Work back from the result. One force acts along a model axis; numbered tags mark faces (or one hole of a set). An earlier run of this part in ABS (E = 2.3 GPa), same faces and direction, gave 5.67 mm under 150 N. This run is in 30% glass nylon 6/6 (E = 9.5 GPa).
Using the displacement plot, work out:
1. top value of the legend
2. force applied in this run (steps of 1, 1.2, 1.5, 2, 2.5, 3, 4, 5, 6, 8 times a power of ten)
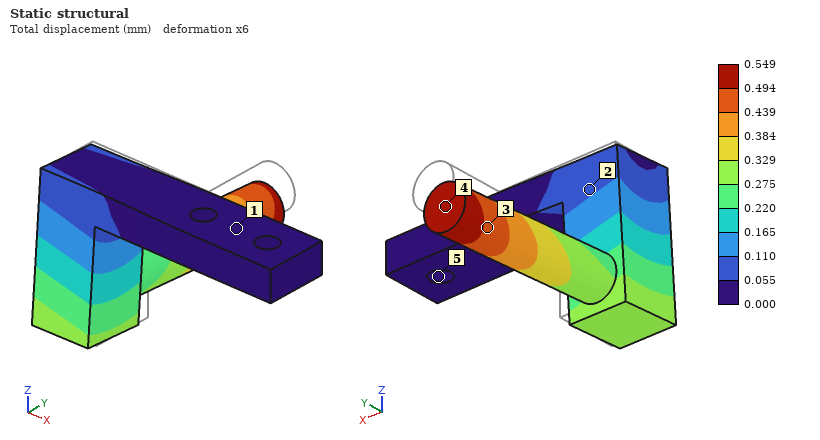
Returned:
0.549 mm
60 N
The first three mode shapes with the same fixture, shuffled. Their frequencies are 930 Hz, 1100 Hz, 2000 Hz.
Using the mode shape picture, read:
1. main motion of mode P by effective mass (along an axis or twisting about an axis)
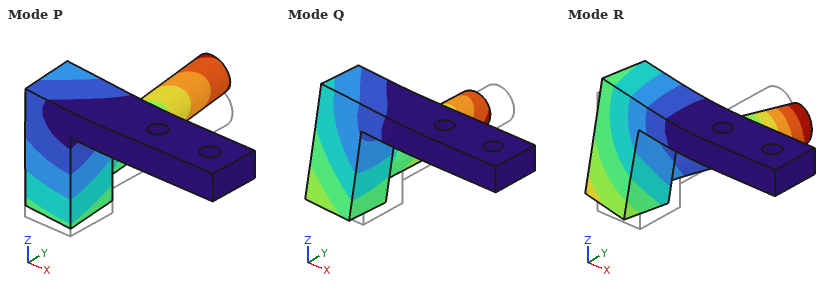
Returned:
along Z
